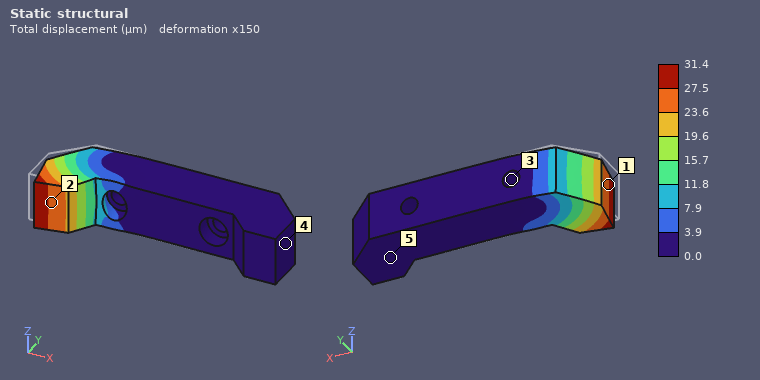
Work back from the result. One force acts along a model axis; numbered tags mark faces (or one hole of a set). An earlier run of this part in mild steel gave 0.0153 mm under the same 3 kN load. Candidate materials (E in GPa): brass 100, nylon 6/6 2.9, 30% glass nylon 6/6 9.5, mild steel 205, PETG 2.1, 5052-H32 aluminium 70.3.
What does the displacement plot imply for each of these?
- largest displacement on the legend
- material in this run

31.4 µm
brass
